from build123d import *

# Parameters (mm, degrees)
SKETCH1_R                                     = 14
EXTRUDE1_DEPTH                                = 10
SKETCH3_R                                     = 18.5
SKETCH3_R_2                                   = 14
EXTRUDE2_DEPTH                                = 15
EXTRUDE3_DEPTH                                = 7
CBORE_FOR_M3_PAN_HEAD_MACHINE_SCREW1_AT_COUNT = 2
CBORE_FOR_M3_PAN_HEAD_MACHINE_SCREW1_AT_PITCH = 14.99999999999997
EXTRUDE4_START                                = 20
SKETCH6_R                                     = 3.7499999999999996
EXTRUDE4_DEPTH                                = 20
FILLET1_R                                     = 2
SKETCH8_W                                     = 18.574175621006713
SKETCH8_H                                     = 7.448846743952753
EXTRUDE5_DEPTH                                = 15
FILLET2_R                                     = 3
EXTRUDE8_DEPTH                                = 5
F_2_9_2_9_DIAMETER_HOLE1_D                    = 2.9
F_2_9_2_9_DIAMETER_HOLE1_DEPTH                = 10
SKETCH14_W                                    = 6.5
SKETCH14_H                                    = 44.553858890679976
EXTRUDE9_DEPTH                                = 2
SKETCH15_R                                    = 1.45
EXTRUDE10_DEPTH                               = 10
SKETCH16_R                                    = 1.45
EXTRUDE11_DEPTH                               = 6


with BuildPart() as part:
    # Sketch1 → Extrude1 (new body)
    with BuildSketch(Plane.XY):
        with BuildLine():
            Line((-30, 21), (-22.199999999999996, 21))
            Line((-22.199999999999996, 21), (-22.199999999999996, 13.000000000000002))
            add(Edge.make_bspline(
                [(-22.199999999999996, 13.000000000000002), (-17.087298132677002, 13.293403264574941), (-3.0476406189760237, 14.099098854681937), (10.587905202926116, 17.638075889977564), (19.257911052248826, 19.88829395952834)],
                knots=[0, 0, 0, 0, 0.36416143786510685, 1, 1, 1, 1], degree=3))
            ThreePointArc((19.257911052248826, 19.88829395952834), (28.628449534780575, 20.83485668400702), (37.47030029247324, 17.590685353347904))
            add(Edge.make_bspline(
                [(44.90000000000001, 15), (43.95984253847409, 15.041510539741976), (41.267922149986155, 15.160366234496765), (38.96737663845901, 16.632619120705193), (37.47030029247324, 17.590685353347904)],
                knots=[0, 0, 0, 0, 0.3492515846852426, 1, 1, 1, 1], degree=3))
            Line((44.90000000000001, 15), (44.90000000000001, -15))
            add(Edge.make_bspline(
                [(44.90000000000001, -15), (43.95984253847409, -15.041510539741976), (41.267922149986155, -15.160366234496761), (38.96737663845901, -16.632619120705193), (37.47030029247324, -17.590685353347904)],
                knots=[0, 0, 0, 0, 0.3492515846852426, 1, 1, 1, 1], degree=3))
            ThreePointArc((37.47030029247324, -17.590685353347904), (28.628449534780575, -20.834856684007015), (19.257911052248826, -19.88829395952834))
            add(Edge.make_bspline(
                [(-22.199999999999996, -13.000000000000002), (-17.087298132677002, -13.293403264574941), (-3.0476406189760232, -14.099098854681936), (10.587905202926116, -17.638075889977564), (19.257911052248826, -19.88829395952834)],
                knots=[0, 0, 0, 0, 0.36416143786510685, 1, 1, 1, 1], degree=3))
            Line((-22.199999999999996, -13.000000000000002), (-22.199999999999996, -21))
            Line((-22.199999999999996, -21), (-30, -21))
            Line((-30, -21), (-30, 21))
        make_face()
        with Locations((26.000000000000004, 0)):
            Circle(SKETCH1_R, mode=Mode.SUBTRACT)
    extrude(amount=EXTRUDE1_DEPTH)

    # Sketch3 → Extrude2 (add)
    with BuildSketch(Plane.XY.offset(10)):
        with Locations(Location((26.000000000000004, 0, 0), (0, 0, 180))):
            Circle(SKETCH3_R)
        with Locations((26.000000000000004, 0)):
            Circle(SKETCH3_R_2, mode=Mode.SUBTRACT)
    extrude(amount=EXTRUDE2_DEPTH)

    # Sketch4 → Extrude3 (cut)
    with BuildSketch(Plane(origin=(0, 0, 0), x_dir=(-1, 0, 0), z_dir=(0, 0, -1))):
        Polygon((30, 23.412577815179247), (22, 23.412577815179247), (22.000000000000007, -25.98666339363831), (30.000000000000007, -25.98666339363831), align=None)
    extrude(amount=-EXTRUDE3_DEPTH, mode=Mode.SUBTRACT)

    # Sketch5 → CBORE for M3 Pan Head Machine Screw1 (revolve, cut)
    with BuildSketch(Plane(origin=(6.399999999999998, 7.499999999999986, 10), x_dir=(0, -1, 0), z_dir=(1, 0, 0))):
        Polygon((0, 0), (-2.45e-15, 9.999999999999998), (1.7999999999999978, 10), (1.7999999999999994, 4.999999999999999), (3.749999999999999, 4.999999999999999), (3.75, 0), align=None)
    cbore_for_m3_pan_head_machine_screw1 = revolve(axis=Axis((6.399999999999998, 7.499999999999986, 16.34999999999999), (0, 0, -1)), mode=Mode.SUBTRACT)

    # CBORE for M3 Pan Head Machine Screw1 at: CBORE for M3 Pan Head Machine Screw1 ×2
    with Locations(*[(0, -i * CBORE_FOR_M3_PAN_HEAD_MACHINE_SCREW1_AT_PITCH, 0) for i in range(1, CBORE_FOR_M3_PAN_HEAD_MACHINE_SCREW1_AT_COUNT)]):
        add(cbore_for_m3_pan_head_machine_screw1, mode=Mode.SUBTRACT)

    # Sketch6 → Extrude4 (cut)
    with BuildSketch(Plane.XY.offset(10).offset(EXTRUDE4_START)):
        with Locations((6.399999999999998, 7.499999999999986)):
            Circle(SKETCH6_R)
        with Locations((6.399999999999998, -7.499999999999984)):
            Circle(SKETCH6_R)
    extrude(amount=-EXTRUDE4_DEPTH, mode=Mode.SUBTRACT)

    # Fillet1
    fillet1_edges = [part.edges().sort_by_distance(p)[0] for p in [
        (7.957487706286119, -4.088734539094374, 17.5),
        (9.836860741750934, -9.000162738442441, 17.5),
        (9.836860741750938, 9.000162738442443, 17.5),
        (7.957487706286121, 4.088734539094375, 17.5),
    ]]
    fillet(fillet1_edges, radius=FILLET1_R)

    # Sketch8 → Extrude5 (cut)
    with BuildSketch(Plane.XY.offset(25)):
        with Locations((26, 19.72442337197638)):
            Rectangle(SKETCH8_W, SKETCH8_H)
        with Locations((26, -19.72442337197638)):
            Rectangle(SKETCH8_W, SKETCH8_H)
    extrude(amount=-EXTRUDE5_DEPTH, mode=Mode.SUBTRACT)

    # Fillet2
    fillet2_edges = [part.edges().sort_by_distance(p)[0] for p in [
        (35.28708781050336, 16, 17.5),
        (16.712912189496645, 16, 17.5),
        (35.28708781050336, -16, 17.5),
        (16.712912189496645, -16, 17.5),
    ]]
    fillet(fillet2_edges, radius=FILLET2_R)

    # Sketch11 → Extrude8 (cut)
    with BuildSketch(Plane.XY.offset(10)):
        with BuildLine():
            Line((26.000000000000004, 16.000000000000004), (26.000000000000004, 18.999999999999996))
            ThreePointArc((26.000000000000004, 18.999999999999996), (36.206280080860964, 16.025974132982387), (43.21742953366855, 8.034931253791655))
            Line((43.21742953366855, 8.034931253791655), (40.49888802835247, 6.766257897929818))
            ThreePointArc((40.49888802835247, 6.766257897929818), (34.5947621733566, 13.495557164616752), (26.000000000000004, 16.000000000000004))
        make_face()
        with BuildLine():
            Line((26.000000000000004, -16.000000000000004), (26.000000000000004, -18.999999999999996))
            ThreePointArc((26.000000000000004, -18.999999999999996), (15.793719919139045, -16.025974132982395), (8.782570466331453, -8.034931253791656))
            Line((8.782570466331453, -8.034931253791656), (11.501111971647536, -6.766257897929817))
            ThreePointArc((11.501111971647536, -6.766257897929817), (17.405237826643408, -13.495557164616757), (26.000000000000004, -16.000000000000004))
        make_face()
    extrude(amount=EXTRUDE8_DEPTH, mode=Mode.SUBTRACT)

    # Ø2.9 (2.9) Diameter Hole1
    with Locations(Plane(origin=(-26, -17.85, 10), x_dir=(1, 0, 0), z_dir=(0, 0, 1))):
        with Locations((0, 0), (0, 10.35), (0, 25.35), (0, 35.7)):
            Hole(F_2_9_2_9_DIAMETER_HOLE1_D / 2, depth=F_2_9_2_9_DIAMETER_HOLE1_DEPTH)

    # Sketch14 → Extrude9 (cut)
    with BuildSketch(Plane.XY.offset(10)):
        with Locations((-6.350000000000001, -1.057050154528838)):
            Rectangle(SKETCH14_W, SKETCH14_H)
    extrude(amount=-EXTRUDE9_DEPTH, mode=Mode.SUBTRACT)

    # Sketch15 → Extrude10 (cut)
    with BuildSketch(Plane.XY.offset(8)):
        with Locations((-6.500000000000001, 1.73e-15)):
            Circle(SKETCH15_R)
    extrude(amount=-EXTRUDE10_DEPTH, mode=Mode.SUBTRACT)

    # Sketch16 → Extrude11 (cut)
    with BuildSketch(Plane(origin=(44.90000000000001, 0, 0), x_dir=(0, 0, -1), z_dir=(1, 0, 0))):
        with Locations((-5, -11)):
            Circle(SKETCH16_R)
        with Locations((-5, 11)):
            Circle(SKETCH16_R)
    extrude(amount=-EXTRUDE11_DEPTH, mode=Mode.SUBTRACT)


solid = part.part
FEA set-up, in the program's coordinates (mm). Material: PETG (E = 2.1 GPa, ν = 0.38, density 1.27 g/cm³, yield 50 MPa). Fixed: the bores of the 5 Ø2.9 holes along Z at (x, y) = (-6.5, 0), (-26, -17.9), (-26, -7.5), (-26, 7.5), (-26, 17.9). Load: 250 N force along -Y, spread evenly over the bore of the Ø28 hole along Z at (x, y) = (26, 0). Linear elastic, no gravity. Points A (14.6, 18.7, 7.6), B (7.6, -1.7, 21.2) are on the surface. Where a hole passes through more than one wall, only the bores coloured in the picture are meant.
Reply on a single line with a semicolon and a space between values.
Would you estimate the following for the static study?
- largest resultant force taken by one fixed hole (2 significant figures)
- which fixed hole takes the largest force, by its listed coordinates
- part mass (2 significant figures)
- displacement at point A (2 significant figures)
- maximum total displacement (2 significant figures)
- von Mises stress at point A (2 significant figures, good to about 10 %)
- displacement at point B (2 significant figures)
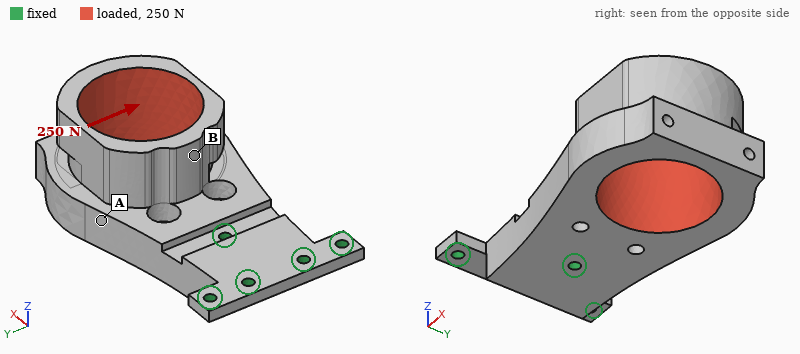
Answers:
500 N; (-6.5, 0); 28 g; 0.42 mm; 0.99 mm; 5.4 MPa; 0.41 mm
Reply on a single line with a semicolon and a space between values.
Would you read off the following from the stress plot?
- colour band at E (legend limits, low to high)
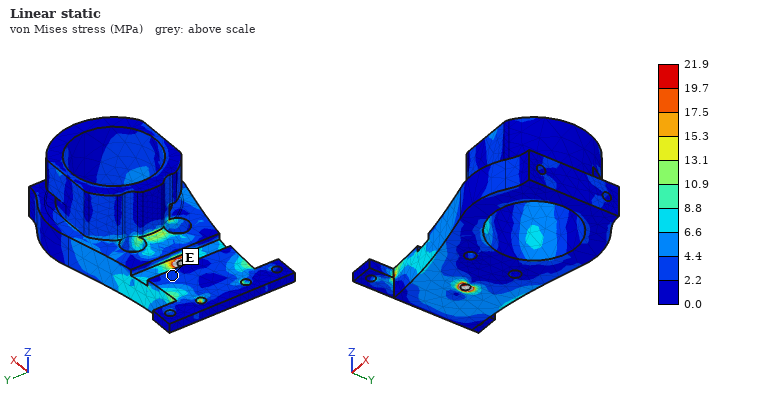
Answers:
2.2 to 4.4 MPa
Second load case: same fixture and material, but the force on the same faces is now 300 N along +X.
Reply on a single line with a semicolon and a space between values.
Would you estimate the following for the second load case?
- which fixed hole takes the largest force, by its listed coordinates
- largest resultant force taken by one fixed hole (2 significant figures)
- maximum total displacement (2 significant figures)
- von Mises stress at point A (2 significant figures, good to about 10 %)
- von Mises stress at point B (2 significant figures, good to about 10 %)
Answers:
(-6.5, 0); 220 N; 0.97 mm; 3.2 MPa; 1.9 MPa
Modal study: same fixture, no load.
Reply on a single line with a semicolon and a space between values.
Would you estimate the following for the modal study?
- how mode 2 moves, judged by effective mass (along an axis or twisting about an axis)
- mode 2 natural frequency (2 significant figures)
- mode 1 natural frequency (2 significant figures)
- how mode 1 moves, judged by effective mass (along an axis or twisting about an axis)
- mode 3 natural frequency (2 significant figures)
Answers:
along Y; 750 Hz; 470 Hz; along Z; 1100 Hz
